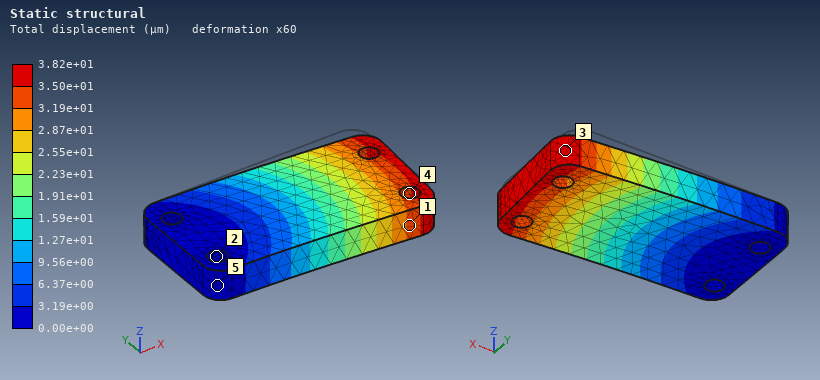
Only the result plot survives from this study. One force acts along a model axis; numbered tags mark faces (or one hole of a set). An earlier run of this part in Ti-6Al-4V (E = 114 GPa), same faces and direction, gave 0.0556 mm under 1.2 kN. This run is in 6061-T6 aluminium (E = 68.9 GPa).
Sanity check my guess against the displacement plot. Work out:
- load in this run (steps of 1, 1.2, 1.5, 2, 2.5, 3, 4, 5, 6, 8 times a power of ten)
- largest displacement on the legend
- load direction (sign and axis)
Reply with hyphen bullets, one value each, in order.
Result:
- 500 N
- 3.82e+01 µm
- -Y
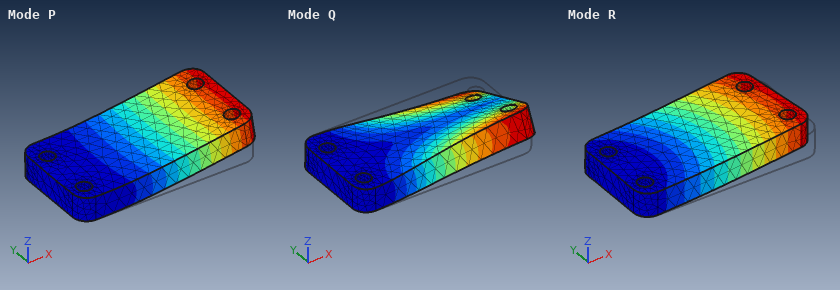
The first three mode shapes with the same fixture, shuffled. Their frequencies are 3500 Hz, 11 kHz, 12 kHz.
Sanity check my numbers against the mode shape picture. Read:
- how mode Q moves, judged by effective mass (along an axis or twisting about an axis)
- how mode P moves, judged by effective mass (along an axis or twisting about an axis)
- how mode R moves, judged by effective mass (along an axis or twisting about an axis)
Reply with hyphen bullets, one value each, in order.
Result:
- twisting about X
- along Z
- along Y
